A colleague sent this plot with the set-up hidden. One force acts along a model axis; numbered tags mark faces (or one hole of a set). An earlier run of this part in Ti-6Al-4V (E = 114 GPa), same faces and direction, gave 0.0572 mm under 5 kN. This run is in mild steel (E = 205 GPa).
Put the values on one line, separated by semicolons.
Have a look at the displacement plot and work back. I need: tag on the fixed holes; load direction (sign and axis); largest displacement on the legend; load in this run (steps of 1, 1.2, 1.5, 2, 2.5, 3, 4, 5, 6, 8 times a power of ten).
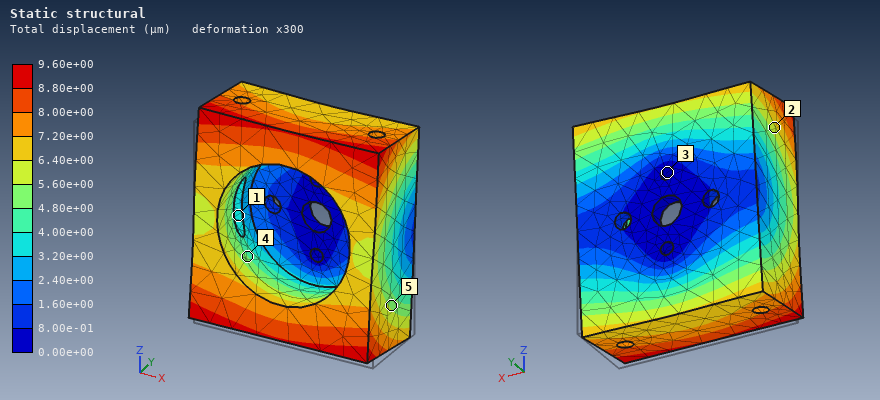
3; +Z; 9.60e+00 µm; 1.5 kN
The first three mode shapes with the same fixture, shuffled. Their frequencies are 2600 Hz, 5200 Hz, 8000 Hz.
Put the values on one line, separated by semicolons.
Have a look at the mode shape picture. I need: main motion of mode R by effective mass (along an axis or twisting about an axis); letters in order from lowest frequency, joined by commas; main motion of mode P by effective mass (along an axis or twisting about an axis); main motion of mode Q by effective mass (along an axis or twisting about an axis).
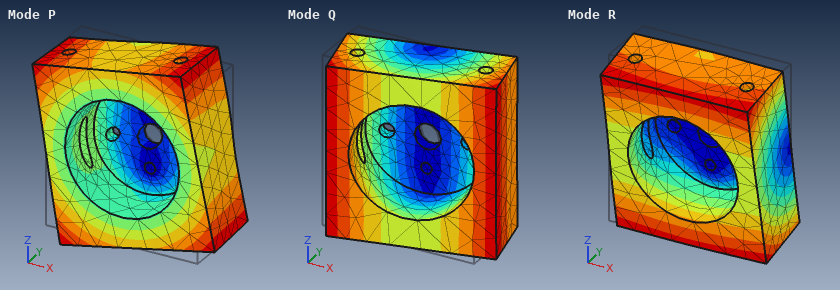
along Z; Q, R, P; twisting about Y; along X
